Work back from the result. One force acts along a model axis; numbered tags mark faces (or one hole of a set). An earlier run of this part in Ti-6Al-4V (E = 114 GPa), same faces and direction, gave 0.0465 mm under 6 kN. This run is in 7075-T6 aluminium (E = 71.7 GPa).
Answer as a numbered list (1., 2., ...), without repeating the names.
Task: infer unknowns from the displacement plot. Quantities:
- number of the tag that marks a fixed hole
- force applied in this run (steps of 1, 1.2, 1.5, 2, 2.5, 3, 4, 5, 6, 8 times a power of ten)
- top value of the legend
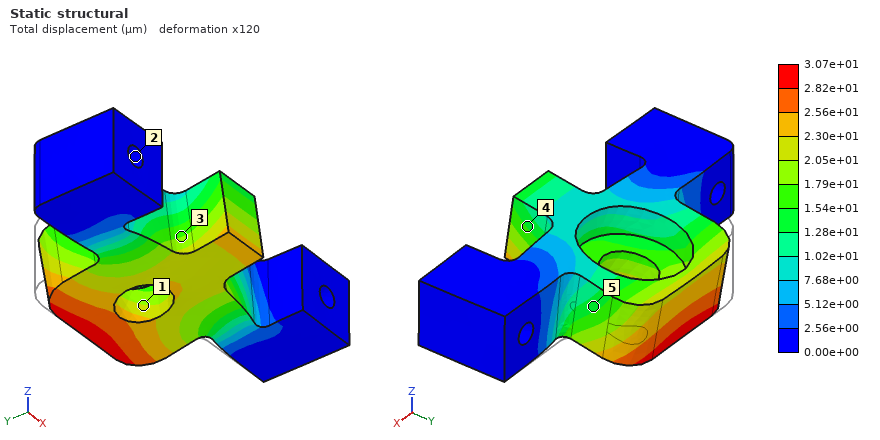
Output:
1. 2
2. 2.5 kN
3. 3.07e+01 µm
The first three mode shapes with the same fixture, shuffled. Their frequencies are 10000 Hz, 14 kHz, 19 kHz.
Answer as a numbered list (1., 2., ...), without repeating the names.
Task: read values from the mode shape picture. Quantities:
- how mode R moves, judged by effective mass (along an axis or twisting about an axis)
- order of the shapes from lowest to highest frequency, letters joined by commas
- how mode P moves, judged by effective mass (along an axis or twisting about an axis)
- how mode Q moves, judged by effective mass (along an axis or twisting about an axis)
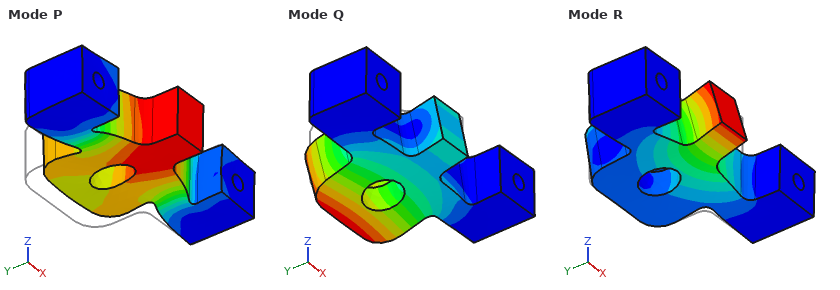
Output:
1. along Z
2. Q, R, P
3. along Y
4. along Z
